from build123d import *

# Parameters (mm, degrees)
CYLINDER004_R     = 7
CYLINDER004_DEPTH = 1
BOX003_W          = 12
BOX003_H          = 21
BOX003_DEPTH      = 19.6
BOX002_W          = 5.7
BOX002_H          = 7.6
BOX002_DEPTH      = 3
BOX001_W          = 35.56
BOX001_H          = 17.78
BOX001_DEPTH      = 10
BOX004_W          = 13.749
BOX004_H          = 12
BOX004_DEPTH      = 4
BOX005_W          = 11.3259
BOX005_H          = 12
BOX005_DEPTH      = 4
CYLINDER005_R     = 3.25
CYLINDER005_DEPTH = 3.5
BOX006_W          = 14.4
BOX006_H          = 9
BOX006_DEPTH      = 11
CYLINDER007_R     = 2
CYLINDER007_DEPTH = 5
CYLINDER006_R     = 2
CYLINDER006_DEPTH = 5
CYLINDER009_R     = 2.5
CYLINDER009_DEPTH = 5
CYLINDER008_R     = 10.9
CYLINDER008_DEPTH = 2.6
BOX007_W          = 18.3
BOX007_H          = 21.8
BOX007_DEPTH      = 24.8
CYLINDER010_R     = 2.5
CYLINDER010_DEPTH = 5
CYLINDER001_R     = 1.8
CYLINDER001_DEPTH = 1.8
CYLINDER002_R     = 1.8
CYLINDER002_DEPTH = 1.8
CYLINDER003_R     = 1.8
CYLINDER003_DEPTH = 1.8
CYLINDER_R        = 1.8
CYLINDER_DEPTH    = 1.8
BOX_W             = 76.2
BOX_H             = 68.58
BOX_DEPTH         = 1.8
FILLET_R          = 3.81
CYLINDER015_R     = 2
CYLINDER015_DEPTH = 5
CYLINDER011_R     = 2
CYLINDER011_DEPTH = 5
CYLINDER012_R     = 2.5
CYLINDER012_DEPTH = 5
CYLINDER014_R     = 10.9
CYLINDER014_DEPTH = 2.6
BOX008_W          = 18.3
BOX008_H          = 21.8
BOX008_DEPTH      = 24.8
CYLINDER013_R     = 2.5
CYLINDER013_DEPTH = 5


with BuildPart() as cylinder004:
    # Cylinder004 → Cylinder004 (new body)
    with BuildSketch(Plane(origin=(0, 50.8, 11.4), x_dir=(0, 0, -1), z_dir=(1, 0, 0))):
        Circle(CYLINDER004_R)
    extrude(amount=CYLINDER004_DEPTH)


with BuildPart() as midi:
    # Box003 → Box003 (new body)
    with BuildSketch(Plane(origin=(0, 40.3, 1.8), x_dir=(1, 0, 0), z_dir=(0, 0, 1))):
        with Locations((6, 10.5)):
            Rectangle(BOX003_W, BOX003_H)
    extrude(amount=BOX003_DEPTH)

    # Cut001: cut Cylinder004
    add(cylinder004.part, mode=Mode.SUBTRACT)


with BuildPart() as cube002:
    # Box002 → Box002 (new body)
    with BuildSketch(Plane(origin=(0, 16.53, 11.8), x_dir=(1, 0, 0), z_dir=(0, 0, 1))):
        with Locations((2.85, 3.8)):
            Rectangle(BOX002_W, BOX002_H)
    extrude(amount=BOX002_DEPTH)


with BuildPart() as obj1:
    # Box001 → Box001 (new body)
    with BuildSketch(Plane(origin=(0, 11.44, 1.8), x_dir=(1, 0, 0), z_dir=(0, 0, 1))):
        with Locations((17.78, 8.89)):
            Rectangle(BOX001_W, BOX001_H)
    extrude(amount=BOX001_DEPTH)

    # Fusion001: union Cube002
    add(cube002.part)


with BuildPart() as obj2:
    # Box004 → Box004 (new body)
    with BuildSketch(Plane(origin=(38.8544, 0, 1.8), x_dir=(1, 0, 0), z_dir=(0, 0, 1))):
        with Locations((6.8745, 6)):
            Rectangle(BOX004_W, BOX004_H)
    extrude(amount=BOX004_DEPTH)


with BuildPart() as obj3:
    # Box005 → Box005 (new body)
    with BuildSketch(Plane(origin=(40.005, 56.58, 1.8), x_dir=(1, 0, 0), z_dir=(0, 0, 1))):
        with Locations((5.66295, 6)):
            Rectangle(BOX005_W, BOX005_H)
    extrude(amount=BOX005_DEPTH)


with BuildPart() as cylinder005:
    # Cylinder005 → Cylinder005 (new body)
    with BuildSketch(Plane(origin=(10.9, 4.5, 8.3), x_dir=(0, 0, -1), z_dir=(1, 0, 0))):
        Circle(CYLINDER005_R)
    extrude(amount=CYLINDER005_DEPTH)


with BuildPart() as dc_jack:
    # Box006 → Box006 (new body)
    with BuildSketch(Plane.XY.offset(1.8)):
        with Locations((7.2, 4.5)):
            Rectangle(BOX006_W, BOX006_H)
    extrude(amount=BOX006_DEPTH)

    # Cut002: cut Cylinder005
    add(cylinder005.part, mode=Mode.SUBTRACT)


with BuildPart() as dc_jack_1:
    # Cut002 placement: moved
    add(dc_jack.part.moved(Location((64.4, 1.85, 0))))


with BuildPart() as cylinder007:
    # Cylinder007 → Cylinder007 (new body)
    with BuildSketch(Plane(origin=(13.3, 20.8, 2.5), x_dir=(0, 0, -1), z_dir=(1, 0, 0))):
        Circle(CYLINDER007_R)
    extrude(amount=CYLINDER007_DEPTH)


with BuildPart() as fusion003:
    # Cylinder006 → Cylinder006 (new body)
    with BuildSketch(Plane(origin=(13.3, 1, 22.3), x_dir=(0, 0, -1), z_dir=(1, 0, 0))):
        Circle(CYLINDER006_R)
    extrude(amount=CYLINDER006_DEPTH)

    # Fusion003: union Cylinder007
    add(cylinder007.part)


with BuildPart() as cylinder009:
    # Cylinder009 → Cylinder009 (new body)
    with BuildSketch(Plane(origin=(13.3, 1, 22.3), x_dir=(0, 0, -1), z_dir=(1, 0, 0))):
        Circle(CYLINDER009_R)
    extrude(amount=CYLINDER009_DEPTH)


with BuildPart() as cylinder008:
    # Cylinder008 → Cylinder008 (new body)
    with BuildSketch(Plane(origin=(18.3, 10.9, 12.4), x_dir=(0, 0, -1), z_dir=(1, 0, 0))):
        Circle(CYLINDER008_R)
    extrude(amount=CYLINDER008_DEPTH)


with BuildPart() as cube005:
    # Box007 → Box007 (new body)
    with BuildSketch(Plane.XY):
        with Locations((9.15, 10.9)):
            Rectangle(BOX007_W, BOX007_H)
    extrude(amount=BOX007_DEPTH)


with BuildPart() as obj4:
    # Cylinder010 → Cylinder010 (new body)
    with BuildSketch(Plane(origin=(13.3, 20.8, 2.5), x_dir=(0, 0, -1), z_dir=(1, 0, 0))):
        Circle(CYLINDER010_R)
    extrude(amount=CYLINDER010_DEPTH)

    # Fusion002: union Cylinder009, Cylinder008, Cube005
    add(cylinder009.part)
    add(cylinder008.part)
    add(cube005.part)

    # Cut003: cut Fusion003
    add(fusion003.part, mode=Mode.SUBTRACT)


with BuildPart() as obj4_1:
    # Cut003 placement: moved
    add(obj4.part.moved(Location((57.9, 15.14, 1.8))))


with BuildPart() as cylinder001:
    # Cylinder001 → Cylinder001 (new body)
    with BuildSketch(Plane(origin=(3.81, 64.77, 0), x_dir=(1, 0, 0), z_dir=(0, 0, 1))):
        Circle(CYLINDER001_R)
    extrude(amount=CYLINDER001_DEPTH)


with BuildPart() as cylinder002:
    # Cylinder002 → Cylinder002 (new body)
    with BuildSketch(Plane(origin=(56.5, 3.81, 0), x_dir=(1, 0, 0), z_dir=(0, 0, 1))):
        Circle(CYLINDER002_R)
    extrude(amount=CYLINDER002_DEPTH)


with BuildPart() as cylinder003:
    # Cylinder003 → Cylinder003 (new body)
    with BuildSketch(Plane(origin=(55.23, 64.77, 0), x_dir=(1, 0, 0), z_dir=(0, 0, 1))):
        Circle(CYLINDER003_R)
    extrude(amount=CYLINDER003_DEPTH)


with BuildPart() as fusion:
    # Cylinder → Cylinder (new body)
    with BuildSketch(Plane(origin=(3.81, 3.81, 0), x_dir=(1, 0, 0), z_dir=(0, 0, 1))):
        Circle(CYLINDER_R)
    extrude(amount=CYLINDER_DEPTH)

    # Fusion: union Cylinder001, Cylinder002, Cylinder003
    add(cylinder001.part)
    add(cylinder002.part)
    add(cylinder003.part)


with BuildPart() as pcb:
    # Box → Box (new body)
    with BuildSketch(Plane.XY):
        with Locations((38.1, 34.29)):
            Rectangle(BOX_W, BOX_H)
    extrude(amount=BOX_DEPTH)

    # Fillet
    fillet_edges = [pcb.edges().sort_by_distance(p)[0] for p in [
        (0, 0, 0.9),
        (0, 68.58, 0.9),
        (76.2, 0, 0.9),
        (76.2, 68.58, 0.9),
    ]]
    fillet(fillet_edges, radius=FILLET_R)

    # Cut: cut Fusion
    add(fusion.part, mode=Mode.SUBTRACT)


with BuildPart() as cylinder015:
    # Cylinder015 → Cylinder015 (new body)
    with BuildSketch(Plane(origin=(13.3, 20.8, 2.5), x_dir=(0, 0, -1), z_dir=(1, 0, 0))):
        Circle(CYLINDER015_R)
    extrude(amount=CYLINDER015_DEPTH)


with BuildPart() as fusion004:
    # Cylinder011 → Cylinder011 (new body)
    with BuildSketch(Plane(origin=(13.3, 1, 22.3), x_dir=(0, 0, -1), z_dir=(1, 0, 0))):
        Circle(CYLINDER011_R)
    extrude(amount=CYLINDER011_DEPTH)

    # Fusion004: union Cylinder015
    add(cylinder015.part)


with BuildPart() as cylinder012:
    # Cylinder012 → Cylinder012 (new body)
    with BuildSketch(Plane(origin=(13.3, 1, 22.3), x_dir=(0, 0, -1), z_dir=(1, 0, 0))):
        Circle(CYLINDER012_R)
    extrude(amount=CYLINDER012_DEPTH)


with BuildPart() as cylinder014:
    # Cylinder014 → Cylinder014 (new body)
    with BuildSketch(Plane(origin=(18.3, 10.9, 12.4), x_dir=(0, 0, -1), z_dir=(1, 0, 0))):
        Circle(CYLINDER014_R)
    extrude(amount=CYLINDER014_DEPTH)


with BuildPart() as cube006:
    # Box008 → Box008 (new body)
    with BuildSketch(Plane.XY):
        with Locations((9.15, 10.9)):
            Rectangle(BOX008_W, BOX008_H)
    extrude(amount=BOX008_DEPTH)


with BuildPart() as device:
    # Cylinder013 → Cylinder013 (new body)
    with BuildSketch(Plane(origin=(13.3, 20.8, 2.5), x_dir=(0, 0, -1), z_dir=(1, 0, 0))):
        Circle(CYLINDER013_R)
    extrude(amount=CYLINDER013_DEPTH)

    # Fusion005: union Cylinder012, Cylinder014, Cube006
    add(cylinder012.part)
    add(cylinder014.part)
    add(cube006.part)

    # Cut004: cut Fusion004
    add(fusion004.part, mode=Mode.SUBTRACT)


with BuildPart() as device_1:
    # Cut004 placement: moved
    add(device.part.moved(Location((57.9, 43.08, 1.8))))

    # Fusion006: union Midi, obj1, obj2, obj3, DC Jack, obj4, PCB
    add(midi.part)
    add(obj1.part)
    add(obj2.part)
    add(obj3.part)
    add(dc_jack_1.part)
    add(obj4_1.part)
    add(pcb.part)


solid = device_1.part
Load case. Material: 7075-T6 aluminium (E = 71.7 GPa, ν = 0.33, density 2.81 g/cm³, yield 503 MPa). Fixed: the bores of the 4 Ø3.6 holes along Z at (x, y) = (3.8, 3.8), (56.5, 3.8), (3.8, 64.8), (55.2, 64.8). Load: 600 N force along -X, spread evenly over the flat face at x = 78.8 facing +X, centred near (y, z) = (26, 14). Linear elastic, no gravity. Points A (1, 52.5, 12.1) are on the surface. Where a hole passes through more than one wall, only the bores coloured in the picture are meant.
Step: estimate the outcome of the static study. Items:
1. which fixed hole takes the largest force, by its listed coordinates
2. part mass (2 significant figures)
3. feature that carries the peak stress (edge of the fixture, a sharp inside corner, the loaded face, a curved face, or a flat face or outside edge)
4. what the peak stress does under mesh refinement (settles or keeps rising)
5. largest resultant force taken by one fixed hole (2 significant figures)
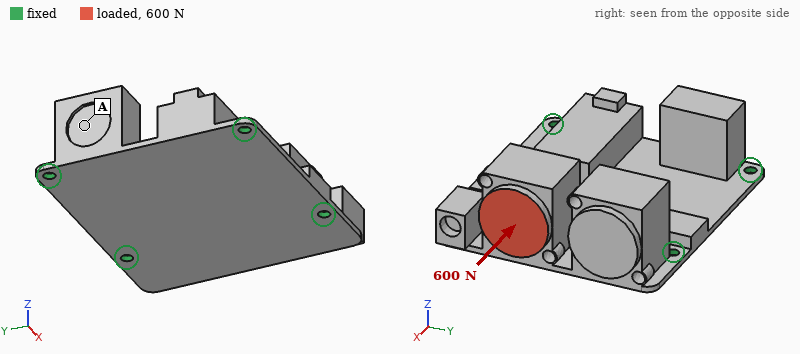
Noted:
(56.5, 3.8)
130 g
edge of the fixture
keeps rising
230 N
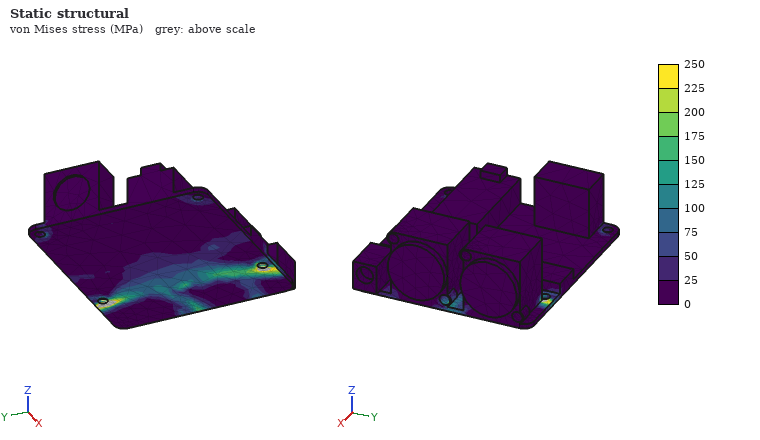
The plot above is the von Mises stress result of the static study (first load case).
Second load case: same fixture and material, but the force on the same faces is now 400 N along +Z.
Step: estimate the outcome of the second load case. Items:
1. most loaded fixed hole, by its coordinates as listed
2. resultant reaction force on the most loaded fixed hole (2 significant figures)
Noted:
(56.5, 3.8)
310 N
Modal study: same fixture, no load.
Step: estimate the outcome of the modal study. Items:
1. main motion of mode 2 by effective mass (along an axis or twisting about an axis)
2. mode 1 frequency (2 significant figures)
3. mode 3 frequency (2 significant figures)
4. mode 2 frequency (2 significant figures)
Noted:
along Z
560 Hz
1700 Hz
1100 Hz
